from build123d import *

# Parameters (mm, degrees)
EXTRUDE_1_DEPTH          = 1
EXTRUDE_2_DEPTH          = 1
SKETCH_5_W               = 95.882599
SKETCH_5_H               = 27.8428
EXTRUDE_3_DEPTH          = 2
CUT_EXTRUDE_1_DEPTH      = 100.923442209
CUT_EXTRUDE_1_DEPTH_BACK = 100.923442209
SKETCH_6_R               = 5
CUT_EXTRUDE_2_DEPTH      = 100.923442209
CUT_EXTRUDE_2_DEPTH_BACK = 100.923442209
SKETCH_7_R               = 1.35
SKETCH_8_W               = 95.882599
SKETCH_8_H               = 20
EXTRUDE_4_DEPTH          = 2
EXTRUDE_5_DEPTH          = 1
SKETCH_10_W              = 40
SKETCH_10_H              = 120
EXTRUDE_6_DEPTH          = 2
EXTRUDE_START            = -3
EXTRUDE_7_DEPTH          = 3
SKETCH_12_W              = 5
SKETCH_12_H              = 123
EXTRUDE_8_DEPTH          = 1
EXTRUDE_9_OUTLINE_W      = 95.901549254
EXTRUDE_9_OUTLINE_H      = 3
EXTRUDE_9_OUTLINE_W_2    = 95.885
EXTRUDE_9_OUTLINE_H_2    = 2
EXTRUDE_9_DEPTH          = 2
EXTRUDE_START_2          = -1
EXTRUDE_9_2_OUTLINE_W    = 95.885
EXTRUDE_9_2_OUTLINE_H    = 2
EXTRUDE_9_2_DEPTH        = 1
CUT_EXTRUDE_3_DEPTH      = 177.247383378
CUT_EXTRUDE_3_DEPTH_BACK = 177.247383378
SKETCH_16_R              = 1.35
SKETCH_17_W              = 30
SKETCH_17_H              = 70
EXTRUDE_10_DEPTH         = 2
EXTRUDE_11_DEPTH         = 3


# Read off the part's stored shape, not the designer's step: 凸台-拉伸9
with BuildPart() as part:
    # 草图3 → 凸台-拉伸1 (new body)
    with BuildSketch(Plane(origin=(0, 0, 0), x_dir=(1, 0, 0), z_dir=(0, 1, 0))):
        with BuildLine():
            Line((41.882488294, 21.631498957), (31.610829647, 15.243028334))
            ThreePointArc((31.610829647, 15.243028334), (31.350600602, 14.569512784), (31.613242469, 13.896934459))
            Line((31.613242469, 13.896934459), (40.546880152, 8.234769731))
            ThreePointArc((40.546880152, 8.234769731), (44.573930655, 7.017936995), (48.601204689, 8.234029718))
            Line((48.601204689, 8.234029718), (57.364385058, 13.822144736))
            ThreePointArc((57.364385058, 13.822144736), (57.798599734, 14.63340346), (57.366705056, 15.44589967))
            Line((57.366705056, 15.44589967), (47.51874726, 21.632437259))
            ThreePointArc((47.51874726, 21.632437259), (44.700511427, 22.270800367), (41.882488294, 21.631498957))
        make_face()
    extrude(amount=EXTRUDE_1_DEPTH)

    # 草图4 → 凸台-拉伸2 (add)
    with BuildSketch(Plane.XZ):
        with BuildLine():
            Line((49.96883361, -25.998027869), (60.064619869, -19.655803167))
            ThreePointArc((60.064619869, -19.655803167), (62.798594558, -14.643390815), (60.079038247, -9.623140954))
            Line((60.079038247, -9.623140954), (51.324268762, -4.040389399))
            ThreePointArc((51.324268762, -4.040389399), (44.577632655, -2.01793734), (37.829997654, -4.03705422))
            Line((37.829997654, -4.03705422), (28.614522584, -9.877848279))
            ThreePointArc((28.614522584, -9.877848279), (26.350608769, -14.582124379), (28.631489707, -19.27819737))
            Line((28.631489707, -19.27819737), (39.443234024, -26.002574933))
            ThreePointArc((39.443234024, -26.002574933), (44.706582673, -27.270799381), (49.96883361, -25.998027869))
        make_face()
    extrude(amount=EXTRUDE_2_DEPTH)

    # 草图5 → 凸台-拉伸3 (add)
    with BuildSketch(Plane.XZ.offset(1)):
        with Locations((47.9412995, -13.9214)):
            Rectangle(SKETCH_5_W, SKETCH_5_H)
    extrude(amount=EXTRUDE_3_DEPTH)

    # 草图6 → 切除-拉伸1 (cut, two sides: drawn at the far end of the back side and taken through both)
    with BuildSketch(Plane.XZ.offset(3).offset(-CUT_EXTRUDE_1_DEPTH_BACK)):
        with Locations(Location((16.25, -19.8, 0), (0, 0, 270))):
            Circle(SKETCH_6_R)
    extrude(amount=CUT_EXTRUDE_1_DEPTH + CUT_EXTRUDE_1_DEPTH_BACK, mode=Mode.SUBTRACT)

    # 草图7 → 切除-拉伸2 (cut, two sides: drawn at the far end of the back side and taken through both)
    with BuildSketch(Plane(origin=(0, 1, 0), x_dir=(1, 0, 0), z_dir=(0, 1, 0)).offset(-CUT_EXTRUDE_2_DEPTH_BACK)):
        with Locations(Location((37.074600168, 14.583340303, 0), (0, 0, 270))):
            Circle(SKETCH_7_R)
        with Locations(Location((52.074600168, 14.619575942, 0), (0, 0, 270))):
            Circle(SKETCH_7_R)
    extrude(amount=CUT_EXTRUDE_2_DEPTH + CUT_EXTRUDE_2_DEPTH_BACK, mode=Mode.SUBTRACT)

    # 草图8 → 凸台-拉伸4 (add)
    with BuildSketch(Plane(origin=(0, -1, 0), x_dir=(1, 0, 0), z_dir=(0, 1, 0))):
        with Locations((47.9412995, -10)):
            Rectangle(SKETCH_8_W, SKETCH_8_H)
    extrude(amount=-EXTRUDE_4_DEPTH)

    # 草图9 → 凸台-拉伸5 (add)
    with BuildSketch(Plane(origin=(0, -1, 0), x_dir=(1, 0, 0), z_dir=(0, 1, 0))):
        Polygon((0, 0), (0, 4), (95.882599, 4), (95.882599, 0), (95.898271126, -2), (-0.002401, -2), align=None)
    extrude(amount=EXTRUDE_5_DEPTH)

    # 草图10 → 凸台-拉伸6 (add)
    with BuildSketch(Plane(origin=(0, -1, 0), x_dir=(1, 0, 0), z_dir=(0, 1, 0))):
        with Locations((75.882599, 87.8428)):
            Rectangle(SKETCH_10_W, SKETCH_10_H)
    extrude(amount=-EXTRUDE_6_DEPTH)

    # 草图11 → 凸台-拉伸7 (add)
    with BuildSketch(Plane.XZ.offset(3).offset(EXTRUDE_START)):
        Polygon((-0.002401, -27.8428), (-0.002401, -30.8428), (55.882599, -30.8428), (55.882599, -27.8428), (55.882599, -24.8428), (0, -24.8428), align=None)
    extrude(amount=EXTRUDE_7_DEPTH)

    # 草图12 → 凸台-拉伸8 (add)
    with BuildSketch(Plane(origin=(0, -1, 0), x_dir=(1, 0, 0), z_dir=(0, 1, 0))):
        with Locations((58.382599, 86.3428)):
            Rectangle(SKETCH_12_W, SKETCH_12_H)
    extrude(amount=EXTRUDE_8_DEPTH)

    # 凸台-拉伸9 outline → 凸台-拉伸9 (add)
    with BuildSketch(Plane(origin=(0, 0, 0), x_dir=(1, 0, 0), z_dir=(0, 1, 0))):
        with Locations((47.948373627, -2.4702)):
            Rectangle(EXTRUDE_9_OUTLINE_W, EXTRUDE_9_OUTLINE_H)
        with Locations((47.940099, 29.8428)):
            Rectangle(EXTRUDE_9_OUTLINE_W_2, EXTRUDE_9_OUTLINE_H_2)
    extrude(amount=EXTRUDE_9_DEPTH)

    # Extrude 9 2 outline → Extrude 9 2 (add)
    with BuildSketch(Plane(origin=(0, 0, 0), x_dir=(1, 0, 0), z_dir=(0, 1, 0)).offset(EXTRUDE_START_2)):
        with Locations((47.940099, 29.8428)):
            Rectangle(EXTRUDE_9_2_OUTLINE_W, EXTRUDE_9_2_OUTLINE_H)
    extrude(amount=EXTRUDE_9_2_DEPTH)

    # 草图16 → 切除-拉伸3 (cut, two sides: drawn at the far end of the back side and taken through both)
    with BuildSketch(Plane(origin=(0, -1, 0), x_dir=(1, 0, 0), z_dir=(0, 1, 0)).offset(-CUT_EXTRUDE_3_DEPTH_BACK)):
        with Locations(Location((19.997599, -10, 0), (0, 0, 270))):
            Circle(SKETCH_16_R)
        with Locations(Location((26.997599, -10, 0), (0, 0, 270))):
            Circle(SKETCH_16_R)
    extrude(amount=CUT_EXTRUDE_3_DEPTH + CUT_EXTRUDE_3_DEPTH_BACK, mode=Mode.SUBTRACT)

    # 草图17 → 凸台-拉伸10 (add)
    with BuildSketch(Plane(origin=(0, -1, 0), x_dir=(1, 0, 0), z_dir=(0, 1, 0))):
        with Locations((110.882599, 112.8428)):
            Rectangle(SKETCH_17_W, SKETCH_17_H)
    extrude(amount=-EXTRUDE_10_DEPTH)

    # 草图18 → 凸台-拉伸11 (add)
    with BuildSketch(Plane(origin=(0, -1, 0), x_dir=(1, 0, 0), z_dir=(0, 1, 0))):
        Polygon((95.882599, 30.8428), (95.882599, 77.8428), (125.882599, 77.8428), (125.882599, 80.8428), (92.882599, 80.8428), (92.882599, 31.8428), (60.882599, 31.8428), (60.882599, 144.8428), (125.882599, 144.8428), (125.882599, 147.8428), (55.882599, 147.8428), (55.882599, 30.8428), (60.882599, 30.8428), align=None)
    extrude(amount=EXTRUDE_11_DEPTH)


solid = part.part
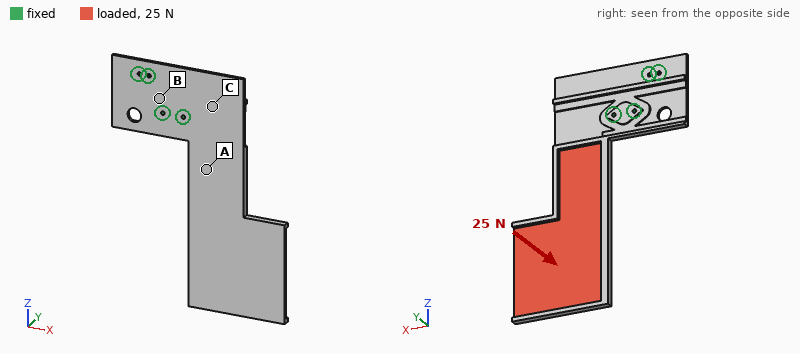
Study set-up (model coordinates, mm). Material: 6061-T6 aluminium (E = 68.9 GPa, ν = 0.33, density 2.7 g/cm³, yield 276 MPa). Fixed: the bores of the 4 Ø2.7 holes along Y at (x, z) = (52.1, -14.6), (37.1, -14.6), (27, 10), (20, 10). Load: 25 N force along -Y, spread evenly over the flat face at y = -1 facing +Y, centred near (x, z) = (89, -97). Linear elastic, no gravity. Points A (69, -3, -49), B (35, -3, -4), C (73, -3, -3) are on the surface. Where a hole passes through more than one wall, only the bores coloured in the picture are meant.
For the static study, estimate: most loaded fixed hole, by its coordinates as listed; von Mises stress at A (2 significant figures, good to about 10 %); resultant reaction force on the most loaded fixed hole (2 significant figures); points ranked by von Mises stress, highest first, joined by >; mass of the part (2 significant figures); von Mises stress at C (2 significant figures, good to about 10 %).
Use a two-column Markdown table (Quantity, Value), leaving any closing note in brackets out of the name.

| Quantity | Value |
|---|---|
| most loaded fixed hole, by its coordinates as listed | (52.1, -14.6) |
| von Mises stress at A | 16 MPa |
| resultant reaction force on the most loaded fixed hole | 72 N |
| points ranked by von Mises stress, highest first, joined by > | A > C > B |
| mass of the part | 78 g |
| von Mises stress at C | 11 MPa |
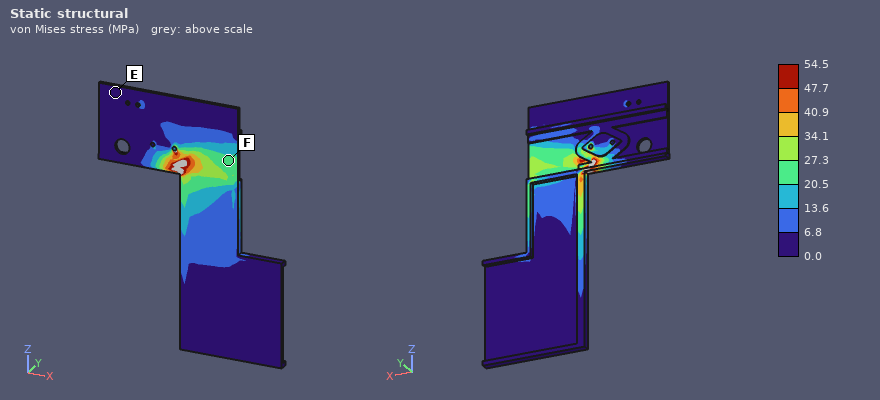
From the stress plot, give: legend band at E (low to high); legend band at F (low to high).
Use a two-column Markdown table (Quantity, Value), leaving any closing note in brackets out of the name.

| Quantity | Value |
|---|---|
| legend band at E | 0.0 to 6.8 MPa |
| legend band at F | 20.5 to 27.3 MPa |
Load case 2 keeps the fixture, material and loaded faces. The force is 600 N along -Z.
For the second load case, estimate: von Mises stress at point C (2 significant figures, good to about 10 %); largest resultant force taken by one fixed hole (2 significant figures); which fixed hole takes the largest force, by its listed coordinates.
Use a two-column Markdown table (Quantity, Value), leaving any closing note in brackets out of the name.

| Quantity | Value |
|---|---|
| von Mises stress at point C | 10 MPa |
| largest resultant force taken by one fixed hole | 990 N |
| which fixed hole takes the largest force, by its listed coordinates | (52.1, -14.6) |
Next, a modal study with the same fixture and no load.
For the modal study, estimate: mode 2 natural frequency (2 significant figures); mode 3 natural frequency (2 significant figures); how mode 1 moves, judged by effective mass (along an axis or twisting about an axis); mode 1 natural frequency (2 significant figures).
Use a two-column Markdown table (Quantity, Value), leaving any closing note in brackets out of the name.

| Quantity | Value |
|---|---|
| mode 2 natural frequency | 360 Hz |
| mode 3 natural frequency | 690 Hz |
| how mode 1 moves, judged by effective mass | along Y |
| mode 1 natural frequency | 100 Hz |
